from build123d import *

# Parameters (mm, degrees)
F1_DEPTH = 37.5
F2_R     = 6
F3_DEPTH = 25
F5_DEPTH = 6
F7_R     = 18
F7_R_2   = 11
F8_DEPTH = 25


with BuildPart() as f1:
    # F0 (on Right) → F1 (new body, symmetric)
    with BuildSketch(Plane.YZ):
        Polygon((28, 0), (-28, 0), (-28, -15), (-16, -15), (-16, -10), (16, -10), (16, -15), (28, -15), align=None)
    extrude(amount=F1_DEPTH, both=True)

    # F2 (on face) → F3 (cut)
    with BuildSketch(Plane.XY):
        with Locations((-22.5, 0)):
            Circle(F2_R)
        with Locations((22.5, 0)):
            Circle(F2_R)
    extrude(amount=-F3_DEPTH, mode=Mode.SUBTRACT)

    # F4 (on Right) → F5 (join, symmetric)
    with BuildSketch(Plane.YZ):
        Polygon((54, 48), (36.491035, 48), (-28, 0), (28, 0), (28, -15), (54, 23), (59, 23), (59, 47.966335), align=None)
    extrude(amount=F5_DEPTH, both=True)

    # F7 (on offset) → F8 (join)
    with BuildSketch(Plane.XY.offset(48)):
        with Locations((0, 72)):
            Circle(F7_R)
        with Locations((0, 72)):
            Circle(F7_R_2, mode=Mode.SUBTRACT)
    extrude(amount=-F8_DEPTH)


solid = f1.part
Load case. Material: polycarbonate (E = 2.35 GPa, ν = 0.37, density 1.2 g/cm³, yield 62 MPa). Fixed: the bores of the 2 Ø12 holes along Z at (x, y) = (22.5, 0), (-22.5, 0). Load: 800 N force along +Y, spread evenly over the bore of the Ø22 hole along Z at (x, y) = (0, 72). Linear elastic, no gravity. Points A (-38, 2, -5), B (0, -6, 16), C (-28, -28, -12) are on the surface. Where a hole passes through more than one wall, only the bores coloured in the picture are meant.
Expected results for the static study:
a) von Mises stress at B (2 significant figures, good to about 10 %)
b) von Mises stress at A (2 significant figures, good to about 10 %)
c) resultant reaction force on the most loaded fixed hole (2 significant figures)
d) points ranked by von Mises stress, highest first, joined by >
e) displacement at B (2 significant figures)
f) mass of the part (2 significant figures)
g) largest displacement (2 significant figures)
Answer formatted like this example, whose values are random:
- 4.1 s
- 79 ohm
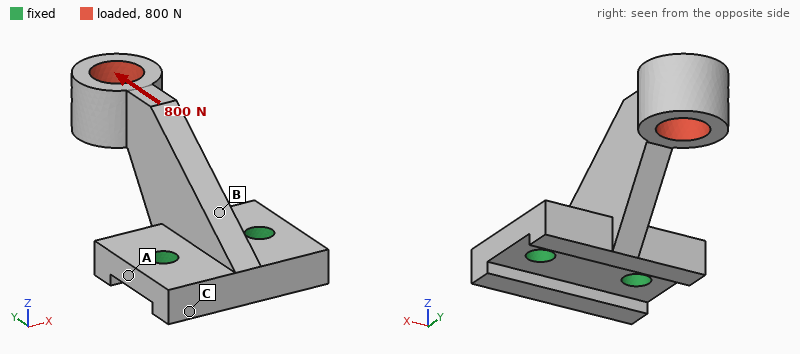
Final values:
- 8.6 MPa
- 5.4 MPa
- 410 N
- B > A > C
- 0.30 mm
- 110 g
- 1.8 mm
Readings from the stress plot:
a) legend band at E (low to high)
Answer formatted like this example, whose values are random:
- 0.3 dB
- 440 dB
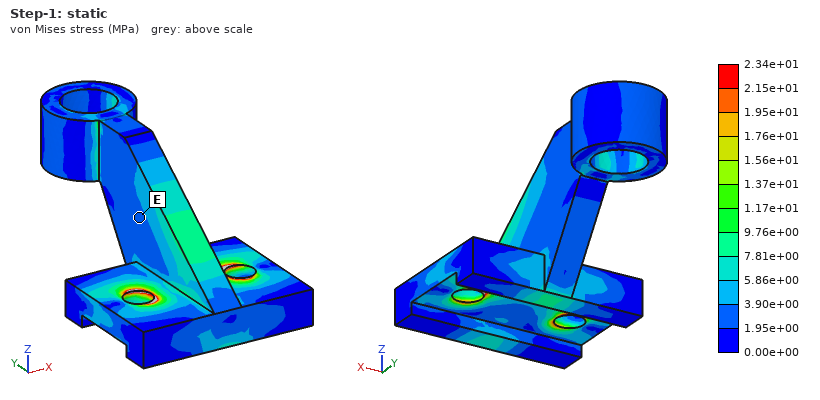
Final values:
- 1.95e+00 to 3.90e+00 MPa
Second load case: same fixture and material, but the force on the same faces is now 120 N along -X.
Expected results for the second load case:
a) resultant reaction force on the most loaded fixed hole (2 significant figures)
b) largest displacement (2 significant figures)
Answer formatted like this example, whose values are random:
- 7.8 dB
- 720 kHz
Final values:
- 220 N
- 1.7 mm
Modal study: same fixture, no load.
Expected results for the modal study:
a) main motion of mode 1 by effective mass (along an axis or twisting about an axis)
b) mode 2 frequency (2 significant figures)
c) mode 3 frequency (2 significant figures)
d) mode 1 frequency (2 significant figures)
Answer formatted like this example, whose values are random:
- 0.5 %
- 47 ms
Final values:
- along X
- 500 Hz
- 980 Hz
- 340 Hz
